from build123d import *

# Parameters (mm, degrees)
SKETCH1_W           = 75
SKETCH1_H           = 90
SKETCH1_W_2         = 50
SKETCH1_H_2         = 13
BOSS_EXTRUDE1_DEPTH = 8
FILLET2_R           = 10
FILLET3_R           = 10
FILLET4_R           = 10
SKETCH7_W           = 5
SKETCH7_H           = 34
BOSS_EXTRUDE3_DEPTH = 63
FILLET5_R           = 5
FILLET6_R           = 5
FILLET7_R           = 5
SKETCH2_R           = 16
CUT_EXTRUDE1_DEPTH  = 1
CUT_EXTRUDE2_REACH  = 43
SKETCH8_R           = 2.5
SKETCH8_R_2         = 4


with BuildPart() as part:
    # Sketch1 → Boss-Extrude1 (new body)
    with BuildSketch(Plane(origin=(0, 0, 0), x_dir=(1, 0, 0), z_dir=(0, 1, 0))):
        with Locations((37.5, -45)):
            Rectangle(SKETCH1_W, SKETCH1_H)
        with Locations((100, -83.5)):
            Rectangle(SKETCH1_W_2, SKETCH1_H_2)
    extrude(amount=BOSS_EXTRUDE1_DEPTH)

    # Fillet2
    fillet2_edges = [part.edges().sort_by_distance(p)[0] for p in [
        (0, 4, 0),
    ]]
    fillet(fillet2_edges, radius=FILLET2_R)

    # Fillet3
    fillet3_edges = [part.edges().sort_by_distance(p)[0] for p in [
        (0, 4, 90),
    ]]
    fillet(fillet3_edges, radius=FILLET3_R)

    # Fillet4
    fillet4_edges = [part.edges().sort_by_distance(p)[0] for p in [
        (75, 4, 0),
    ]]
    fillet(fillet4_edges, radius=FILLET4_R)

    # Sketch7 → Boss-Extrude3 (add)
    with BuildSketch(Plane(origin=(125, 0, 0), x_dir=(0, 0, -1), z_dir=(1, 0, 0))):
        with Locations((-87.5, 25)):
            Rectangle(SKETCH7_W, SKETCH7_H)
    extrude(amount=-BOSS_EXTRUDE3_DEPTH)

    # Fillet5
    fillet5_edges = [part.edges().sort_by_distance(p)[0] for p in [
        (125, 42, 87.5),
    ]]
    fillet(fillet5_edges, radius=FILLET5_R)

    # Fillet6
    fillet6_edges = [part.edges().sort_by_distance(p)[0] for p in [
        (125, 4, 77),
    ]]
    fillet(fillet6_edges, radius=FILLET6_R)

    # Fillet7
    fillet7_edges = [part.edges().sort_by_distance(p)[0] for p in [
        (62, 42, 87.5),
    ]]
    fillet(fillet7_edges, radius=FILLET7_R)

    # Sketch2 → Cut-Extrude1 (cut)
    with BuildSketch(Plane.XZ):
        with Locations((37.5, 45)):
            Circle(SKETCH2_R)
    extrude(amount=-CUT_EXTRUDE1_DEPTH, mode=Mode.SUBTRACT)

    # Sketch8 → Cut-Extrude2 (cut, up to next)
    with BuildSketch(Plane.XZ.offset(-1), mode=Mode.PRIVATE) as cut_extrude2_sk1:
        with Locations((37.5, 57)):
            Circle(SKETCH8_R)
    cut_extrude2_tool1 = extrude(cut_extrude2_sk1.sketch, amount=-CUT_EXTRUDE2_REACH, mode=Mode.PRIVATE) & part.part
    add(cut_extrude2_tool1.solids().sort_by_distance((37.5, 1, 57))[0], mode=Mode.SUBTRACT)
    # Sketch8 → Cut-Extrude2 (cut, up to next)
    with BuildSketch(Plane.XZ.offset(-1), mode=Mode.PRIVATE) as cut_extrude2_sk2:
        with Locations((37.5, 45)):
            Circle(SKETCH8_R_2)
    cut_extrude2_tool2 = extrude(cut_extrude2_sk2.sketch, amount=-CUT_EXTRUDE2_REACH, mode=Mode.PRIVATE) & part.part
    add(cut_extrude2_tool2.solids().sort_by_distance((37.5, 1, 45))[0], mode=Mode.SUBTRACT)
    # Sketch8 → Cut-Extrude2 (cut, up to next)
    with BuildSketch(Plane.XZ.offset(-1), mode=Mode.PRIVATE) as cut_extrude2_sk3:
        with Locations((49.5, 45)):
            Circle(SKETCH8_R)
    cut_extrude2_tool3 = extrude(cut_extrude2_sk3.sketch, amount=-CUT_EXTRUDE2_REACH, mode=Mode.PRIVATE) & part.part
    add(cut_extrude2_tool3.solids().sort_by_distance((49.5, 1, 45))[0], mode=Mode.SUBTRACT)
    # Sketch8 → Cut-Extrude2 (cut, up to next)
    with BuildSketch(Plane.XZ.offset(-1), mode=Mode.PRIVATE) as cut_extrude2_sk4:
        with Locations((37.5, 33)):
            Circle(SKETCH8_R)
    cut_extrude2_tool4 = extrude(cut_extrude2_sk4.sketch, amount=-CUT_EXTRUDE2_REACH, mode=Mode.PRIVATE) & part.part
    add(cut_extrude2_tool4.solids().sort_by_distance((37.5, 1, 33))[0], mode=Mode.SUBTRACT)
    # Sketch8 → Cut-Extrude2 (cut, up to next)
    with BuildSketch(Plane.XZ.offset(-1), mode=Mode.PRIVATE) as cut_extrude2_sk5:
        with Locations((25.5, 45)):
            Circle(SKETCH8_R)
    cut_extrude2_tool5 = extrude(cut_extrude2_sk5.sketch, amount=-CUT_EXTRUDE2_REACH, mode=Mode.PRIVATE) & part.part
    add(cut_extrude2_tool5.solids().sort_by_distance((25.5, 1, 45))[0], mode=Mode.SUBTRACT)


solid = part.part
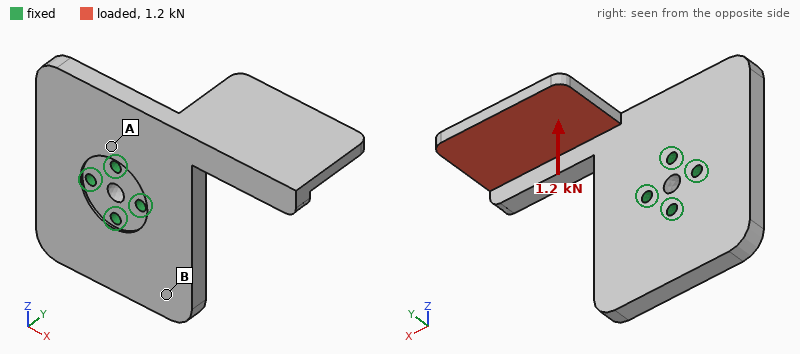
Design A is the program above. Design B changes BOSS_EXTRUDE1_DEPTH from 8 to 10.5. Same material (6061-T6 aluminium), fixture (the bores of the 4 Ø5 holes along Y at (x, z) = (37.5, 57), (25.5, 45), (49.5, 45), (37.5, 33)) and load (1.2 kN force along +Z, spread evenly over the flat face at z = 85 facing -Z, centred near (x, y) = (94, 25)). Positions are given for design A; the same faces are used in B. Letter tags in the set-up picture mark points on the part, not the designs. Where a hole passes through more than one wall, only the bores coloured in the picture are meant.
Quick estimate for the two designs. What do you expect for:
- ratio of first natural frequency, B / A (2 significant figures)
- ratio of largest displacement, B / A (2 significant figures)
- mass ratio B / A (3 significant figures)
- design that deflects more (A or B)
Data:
1.4
0.61
1.25
A
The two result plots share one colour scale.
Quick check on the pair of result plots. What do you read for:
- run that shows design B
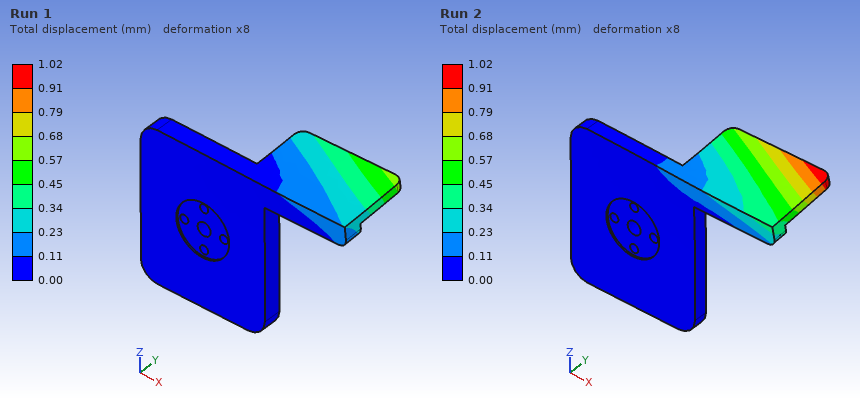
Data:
Run 1
